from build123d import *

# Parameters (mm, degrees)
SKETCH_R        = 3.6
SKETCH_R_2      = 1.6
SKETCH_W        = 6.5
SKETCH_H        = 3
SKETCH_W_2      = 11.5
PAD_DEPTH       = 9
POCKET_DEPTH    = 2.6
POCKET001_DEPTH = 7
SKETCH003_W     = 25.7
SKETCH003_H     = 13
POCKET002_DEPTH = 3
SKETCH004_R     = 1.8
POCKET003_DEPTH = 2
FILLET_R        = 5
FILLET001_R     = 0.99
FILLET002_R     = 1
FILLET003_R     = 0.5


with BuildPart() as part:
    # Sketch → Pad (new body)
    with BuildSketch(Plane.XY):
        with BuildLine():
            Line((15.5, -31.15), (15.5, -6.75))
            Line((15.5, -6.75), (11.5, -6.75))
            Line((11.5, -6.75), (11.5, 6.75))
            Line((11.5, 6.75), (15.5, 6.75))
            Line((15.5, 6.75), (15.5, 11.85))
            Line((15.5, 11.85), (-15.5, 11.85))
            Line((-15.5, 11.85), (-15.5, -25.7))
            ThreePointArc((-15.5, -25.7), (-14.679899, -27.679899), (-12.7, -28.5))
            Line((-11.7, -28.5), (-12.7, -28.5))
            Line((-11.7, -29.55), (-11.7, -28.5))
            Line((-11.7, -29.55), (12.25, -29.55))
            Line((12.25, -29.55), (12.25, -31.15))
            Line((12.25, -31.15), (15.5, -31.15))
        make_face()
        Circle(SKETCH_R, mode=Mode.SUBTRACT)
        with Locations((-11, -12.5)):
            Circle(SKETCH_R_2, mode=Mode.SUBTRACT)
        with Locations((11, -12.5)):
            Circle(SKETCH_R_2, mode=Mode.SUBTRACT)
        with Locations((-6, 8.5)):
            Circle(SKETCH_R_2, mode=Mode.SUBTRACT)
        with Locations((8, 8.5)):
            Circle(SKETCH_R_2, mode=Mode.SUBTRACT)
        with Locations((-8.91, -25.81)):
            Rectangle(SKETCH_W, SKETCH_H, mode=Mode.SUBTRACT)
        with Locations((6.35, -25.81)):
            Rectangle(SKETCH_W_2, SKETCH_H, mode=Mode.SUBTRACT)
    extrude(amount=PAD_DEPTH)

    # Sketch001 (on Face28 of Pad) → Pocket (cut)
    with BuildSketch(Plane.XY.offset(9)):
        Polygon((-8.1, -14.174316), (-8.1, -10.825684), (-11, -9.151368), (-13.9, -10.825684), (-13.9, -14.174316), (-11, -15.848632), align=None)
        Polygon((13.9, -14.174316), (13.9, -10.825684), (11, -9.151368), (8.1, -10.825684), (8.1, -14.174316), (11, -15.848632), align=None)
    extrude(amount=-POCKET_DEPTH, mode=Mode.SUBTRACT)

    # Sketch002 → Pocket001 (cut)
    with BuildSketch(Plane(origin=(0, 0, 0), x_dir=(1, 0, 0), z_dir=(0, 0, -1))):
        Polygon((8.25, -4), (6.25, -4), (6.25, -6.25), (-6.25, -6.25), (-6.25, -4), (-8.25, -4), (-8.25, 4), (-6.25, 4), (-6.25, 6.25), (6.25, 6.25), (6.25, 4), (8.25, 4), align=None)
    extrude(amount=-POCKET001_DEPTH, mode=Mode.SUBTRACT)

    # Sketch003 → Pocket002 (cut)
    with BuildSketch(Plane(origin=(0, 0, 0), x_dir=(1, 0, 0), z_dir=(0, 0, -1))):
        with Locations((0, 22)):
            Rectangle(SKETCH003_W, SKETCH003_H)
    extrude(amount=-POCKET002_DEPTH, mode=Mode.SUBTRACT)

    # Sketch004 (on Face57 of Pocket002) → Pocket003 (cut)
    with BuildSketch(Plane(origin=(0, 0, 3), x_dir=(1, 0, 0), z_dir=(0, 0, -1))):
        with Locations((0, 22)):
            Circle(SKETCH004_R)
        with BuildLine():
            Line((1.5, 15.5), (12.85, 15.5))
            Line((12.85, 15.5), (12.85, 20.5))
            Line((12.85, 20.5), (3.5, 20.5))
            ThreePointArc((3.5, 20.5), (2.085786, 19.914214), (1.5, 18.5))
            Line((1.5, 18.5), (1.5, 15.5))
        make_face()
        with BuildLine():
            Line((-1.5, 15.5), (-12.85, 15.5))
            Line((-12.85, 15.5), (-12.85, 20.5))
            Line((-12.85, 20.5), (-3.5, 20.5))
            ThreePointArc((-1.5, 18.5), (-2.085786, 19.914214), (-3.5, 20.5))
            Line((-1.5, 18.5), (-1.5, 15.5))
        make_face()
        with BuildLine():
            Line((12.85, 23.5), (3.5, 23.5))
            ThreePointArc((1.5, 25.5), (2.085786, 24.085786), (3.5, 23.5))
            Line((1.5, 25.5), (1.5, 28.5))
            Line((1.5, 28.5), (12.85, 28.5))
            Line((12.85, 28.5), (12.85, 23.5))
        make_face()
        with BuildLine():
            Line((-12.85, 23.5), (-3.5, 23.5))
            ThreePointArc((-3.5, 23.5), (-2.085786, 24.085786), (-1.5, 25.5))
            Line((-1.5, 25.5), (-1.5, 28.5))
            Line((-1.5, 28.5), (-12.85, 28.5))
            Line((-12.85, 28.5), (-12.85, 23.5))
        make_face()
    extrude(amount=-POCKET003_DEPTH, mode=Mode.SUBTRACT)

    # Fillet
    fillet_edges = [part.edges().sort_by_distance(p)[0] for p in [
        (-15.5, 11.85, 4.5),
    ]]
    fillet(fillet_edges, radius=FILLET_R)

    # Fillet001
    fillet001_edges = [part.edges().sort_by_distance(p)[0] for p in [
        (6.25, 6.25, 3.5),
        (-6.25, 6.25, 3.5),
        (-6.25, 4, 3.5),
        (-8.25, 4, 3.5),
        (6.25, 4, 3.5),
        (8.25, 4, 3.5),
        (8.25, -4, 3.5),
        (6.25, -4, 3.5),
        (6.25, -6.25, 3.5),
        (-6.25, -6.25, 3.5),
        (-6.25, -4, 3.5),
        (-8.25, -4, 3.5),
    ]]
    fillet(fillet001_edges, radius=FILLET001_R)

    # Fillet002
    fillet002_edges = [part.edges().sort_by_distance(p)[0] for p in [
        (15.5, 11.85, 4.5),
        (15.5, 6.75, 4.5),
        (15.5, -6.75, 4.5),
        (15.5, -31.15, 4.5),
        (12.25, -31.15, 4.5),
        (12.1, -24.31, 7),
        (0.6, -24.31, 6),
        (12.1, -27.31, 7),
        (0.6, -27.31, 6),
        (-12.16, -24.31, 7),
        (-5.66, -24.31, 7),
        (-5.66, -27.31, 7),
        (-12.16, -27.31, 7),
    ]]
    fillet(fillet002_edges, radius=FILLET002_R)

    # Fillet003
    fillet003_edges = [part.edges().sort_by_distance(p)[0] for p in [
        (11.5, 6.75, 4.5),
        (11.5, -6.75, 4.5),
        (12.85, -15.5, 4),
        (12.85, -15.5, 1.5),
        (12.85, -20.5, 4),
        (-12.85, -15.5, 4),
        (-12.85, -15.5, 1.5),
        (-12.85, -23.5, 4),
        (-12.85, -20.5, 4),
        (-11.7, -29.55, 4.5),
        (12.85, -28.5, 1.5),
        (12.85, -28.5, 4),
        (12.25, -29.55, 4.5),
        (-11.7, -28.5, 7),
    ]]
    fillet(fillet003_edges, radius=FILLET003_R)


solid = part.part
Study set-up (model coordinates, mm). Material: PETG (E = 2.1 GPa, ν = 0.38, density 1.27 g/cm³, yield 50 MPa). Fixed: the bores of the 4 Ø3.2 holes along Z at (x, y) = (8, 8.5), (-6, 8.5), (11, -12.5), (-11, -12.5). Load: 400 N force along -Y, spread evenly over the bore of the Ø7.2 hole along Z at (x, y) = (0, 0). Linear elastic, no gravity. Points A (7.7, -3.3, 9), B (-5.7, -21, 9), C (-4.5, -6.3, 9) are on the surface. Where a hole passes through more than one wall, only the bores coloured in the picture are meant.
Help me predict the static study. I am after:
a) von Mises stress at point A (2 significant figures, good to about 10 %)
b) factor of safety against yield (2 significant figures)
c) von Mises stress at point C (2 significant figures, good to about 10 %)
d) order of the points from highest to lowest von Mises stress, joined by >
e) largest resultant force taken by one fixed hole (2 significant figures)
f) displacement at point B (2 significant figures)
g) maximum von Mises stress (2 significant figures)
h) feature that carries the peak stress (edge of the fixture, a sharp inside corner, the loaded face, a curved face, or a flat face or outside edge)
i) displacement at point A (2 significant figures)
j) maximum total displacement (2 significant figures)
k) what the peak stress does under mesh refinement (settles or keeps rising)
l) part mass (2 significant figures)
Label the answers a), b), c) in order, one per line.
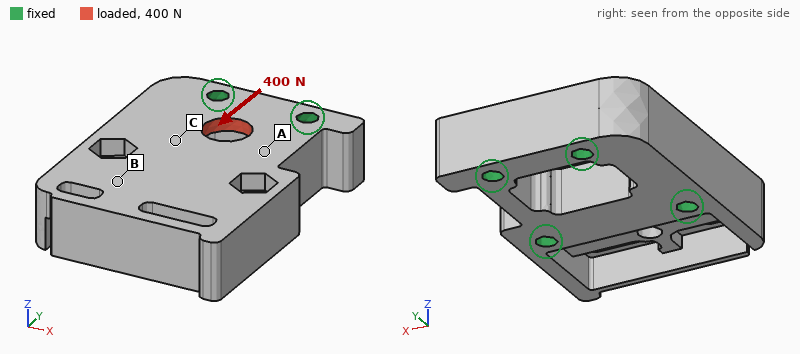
a) 2.7 MPa
b) 3.0
c) 4.9 MPa
d) C > A > B
e) 140 N
f) 16 µm
g) 17 MPa
h) the loaded face
i) 13 µm
j) 45 µm
k) settles
l) 9.6 g
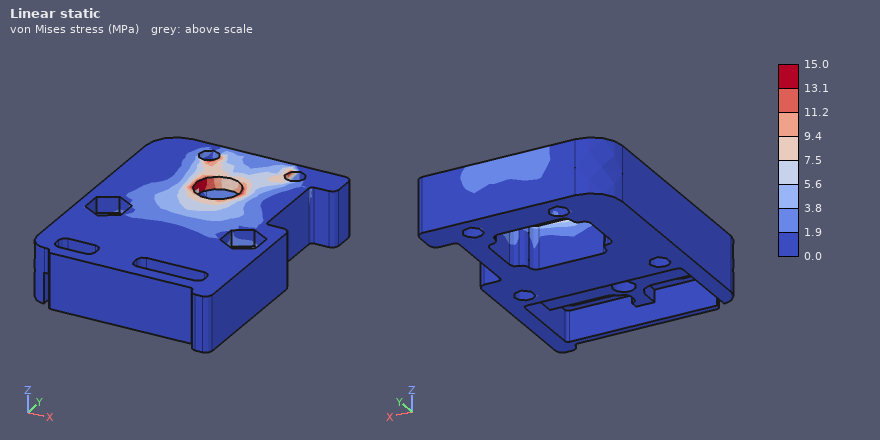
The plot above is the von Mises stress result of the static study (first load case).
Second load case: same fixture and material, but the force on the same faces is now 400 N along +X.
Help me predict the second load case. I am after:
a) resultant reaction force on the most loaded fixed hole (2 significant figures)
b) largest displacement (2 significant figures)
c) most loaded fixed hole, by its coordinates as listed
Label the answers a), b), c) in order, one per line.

a) 120 N
b) 45 µm
c) (-6, 8.5)
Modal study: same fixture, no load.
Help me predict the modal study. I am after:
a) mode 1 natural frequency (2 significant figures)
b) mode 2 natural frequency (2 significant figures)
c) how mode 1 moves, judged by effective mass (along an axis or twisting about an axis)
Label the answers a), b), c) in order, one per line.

a) 3300 Hz
b) 4500 Hz
c) along Z
